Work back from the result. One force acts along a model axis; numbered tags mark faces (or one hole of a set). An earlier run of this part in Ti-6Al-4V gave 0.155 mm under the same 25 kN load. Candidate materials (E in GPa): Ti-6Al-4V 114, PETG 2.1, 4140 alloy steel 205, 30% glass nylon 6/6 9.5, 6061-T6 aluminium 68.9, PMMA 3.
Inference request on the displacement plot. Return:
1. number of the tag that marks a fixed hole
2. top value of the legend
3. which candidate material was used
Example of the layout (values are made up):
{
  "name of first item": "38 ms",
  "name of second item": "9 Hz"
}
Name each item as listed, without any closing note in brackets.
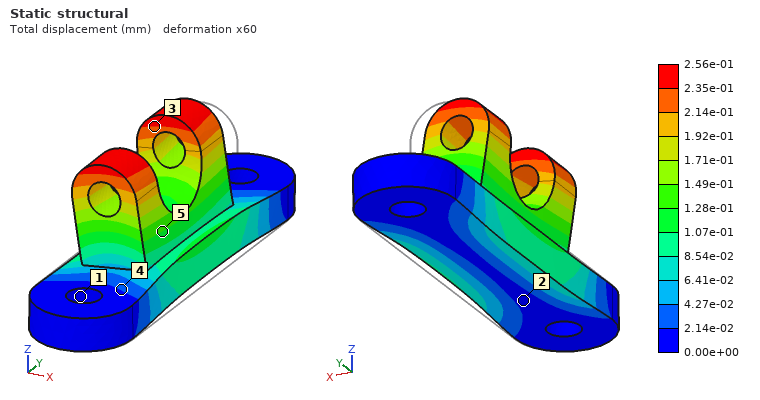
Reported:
{
  "number of the tag that marks a fixed hole": "1",
  "top value of the legend": "2.56e-01 mm",
  "which candidate material was used": "6061-T6 aluminium"
}
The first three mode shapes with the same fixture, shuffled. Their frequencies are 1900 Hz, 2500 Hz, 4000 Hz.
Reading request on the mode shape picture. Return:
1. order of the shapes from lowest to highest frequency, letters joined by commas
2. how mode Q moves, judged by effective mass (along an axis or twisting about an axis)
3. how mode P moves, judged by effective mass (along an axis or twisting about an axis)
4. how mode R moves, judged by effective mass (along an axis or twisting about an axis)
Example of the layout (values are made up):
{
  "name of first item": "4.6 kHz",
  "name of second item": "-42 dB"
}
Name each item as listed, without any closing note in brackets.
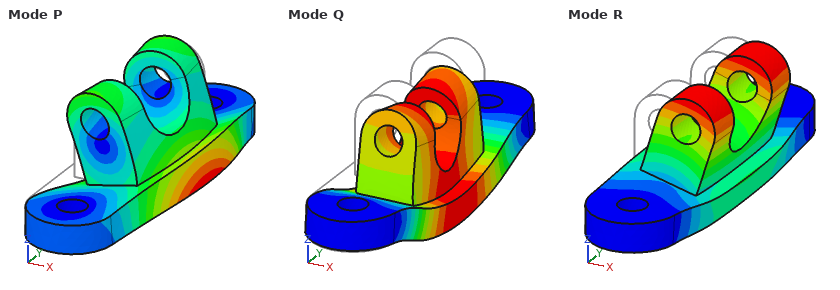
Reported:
{
  "order of the shapes from lowest to highest frequency, letters joined by commas": "R, Q, P",
  "how mode Q moves, judged by effective mass": "along Z",
  "how mode P moves, judged by effective mass": "along X",
  "how mode R moves, judged by effective mass": "along X"
}
